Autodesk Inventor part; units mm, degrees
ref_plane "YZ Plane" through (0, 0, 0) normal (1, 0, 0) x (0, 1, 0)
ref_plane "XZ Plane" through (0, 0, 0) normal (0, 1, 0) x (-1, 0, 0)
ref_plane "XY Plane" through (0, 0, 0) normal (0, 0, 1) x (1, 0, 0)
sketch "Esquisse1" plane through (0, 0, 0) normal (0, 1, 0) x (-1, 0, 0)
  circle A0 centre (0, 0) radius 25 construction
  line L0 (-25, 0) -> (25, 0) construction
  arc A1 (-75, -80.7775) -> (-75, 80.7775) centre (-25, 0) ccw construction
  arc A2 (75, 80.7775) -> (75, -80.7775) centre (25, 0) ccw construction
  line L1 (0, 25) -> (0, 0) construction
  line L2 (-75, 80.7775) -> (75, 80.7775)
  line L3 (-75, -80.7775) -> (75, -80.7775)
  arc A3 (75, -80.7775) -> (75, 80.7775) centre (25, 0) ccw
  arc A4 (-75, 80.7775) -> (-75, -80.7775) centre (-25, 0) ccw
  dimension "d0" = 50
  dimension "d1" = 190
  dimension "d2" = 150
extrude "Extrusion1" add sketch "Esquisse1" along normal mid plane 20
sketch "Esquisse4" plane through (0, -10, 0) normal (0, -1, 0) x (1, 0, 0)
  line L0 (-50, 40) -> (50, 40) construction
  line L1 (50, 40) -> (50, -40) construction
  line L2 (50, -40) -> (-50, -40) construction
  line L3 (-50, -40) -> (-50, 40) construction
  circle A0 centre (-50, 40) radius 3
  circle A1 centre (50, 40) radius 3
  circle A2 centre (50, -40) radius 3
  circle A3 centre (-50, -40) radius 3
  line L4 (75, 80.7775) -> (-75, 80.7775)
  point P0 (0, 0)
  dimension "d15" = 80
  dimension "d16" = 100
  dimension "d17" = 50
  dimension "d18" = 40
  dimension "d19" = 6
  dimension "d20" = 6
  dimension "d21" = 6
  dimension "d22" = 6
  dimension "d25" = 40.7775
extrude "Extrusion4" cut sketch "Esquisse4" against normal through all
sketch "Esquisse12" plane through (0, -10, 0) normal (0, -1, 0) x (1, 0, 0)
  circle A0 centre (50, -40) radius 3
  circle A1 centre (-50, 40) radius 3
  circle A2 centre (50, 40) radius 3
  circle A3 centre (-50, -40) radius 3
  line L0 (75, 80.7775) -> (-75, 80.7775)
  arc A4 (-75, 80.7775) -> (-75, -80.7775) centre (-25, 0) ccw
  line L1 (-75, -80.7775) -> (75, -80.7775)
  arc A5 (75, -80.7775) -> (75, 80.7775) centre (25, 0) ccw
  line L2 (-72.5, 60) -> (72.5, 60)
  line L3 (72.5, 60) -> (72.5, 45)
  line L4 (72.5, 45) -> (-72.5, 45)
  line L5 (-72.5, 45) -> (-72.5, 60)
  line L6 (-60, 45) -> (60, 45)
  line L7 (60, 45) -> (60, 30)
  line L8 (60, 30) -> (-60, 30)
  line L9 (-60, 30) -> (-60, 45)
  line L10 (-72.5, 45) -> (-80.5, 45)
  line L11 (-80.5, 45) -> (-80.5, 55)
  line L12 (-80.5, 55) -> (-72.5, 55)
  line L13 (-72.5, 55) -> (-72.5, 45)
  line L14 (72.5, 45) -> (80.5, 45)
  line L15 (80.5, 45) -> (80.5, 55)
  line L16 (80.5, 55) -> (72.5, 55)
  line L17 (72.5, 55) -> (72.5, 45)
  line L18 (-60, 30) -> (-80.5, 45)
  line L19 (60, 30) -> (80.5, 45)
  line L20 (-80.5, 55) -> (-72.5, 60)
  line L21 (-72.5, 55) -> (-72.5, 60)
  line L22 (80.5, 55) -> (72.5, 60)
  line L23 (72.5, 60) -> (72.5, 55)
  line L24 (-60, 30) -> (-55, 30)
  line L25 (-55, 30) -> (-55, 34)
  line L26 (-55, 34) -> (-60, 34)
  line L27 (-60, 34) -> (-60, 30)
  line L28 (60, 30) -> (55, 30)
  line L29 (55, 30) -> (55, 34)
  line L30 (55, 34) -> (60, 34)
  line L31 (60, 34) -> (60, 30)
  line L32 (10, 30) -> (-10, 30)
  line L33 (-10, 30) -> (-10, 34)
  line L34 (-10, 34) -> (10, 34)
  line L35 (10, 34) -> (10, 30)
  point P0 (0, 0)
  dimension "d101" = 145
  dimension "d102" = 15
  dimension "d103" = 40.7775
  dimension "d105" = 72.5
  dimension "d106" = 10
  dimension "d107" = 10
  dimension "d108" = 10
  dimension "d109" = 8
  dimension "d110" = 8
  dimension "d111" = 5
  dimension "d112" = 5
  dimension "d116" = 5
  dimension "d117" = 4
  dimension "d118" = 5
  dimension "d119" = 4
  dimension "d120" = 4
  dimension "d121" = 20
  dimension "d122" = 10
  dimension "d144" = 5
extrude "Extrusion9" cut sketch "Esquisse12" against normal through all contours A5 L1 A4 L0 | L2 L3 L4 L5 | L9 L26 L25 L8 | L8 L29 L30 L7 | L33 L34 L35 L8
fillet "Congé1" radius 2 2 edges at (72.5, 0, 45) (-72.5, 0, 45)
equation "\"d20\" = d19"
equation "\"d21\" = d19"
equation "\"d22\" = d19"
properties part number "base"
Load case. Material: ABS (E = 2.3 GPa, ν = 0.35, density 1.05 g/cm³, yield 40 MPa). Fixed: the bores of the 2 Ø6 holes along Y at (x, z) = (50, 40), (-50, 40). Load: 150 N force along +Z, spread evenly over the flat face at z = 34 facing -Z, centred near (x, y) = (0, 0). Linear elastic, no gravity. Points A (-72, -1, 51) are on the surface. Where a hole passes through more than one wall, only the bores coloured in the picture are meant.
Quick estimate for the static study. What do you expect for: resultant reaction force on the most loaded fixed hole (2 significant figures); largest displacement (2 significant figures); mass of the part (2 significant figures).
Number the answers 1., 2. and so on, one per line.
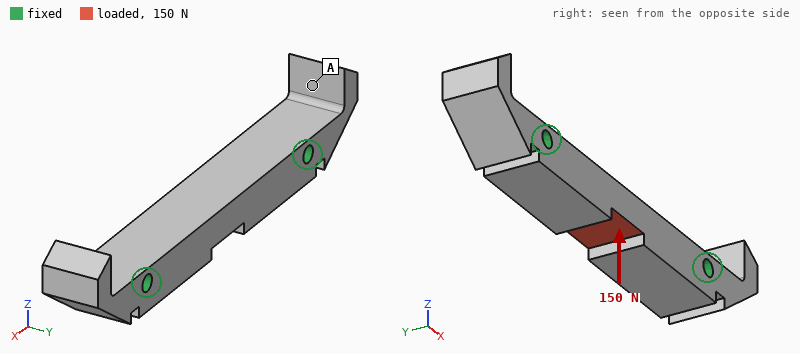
1. 78 N
2. 0.12 mm
3. 45 g
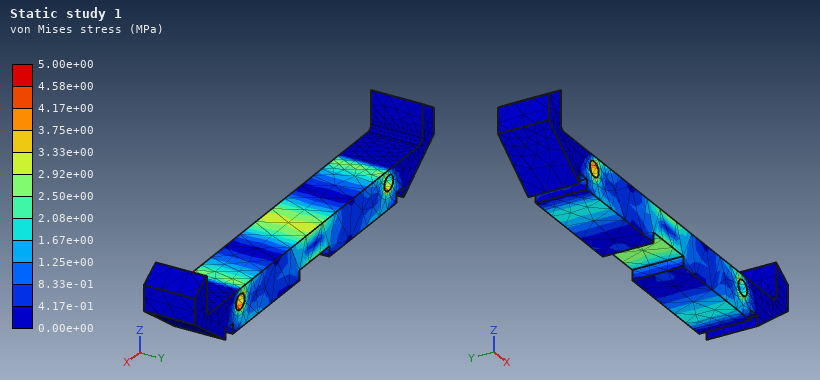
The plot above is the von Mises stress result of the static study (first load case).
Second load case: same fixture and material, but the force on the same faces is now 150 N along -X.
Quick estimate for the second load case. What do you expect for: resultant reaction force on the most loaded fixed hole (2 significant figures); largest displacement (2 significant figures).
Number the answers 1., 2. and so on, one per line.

1. 76 N
2. 8.2 µm
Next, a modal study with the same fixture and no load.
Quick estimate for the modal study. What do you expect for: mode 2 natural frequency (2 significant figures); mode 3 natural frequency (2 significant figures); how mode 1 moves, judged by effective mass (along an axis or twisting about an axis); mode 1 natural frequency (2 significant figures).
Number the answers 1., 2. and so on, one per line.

1. 2000 Hz
2. 2000 Hz
3. along Z
4. 1600 Hz
